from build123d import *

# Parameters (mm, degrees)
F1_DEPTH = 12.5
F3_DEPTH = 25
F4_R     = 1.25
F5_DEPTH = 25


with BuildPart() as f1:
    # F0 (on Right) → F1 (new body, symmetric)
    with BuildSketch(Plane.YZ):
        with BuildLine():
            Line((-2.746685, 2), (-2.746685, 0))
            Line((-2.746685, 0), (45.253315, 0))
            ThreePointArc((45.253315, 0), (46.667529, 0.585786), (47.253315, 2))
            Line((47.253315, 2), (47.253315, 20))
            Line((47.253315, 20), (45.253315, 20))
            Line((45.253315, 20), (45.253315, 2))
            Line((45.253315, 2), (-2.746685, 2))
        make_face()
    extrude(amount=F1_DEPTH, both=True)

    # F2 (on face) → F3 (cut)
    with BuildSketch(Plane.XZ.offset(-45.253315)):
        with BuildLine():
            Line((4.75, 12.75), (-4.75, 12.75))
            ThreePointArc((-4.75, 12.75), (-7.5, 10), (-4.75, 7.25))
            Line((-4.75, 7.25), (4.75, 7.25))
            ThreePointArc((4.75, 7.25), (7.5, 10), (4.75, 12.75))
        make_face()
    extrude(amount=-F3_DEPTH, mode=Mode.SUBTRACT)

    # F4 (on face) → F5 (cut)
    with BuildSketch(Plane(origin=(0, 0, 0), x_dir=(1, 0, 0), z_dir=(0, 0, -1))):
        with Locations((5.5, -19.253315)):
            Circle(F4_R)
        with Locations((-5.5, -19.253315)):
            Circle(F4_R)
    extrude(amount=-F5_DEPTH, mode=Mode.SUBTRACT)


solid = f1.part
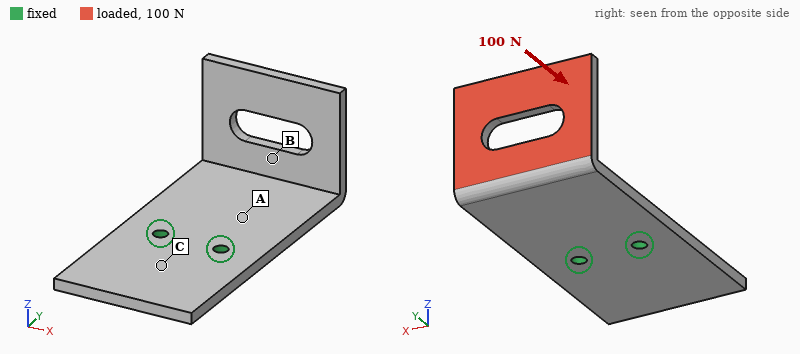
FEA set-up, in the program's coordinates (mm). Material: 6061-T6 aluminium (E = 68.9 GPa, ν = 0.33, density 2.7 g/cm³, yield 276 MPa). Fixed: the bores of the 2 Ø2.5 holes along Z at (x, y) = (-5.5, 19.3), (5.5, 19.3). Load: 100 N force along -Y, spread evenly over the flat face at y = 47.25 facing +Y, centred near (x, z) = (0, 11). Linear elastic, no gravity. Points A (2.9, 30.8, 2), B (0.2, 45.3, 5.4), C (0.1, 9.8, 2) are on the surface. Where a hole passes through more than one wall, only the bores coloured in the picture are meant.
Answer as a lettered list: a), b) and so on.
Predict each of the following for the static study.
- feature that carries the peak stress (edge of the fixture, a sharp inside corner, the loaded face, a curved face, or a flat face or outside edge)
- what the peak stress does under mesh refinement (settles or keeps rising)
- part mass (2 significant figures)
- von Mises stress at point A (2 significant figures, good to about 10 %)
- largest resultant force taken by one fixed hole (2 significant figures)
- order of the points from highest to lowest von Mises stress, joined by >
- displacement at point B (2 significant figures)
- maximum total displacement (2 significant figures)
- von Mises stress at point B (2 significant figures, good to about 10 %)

a) edge of the fixture
b) keeps rising
c) 8.7 g
d) 58 MPa
e) 50 N
f) A > B > C
g) 0.30 mm
h) 0.65 mm
i) 19 MPa
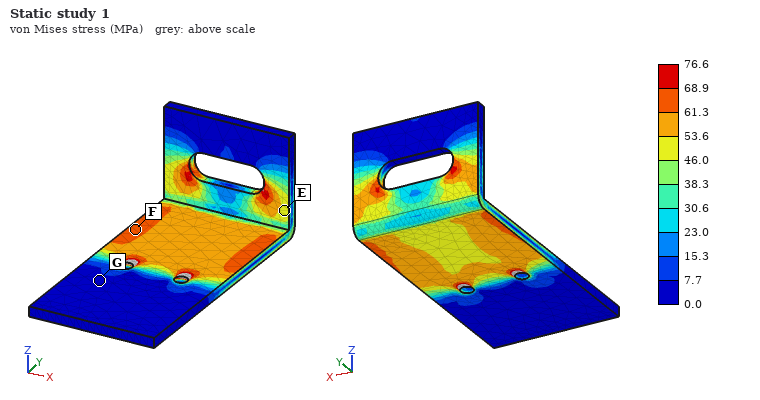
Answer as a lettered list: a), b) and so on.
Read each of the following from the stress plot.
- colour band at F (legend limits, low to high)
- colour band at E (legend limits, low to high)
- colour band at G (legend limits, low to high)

a) 61.3 to 68.9 MPa
b) 46.0 to 53.6 MPa
c) 0.0 to 7.7 MPa
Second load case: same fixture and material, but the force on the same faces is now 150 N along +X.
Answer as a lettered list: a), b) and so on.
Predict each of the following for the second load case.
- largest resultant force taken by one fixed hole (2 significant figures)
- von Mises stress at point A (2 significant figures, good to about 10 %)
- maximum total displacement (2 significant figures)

a) 360 N
b) 79 MPa
c) 0.41 mm
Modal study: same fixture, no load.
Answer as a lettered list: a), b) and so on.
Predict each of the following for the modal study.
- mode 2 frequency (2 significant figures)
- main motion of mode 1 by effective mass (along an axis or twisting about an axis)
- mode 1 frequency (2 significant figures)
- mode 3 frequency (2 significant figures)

a) 2200 Hz
b) along Z
c) 1100 Hz
d) 3100 Hz
